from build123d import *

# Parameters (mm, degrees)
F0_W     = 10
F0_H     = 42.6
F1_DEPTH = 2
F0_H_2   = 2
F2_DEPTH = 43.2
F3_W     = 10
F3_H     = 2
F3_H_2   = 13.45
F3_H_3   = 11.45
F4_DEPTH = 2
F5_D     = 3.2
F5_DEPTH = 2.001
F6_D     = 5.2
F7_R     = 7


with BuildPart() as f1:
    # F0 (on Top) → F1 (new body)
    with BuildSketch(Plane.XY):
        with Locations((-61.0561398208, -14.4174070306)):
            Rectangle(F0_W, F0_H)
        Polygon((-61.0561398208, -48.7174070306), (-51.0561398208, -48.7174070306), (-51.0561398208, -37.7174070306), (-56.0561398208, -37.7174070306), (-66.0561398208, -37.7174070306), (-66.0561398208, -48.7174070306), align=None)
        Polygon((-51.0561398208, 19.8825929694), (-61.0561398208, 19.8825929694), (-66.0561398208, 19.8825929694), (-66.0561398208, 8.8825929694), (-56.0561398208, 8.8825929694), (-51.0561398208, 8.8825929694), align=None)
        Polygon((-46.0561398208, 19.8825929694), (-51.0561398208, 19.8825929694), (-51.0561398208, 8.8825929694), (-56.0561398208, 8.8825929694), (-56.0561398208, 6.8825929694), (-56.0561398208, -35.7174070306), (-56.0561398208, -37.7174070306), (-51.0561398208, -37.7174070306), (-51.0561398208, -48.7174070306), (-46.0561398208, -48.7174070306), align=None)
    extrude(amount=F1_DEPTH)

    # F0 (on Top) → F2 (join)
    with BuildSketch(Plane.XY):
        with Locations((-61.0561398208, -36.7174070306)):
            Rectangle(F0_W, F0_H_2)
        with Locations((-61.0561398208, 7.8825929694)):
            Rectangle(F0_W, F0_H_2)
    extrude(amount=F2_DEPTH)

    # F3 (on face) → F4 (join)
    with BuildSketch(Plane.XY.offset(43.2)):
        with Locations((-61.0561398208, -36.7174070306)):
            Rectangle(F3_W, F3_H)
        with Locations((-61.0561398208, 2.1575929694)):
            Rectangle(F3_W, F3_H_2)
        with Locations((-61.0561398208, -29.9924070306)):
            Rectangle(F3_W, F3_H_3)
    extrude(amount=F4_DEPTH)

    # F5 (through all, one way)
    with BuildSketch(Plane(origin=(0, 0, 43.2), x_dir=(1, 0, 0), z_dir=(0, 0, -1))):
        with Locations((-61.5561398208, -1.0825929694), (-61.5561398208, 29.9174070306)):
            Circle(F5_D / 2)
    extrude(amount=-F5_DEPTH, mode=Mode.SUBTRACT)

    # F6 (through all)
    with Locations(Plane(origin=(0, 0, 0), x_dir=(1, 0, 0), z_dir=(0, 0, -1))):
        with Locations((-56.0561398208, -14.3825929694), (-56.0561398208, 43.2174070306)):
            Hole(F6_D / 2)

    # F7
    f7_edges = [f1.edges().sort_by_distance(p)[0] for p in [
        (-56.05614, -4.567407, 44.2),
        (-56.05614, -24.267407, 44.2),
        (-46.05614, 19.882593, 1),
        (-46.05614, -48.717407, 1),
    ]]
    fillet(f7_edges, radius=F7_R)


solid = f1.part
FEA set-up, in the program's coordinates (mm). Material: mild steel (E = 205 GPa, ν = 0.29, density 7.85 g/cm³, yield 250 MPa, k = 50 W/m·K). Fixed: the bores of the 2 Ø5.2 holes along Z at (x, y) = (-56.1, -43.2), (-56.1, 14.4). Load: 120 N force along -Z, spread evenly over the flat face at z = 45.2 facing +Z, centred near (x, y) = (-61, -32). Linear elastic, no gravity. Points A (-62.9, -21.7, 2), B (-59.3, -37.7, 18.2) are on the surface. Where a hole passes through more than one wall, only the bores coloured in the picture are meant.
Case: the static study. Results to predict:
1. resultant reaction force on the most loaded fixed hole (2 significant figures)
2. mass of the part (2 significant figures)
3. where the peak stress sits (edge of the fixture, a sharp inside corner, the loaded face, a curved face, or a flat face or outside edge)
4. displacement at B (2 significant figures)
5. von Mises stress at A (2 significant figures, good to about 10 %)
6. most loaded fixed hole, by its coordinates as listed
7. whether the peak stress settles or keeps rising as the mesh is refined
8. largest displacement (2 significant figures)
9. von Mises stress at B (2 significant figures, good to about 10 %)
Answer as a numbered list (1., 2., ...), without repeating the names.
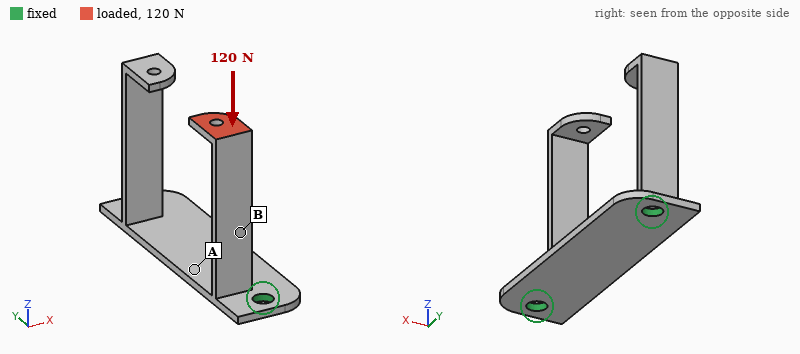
1. 110 N
2. 37 g
3. edge of the fixture
4. 0.093 mm
5. 15 MPa
6. (-56.1, -43.2)
7. keeps rising
8. 0.58 mm
9. 87 MPa
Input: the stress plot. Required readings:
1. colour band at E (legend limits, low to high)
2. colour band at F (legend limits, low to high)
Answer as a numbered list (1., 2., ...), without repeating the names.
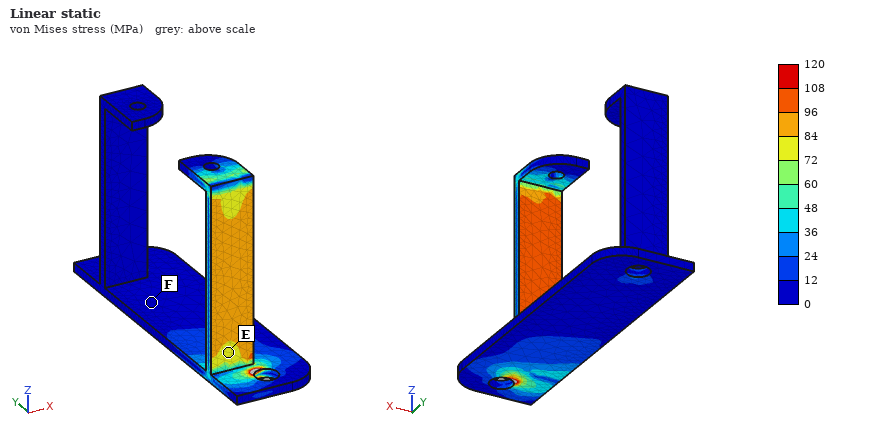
1. 72 to 84 MPa
2. 0 to 12 MPa
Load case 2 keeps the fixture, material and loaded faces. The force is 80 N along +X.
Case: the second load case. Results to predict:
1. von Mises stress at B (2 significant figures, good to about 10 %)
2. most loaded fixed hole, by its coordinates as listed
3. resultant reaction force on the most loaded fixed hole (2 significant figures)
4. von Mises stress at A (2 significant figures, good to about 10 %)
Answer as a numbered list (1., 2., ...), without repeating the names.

1. 57 MPa
2. (-56.1, -43.2)
3. 71 N
4. 33 MPa
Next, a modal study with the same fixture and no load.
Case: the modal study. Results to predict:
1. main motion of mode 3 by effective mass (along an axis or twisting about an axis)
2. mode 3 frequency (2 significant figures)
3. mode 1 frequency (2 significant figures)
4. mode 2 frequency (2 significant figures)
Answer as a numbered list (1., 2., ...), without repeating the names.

1. along X
2. 1400 Hz
3. 570 Hz
4. 590 Hz
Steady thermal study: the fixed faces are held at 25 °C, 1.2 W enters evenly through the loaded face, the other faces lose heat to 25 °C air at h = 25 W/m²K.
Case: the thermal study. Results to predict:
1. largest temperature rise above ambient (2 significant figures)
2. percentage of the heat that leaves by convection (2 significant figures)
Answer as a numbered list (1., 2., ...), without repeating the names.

1. 40 K
2. 54 %
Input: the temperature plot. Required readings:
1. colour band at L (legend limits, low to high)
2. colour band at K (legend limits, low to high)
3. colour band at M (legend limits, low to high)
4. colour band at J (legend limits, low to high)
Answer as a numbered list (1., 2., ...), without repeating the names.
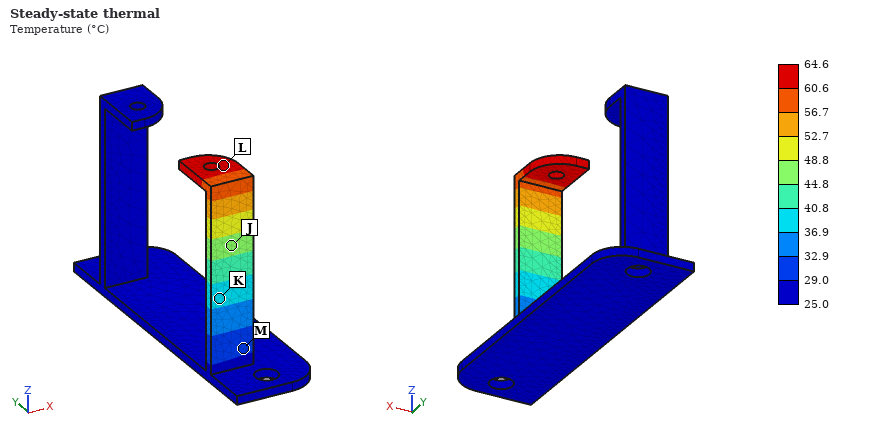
1. 60.6 to 64.6 °C
2. 36.9 to 40.8 °C
3. 29.0 to 32.9 °C
4. 44.8 to 48.8 °C
